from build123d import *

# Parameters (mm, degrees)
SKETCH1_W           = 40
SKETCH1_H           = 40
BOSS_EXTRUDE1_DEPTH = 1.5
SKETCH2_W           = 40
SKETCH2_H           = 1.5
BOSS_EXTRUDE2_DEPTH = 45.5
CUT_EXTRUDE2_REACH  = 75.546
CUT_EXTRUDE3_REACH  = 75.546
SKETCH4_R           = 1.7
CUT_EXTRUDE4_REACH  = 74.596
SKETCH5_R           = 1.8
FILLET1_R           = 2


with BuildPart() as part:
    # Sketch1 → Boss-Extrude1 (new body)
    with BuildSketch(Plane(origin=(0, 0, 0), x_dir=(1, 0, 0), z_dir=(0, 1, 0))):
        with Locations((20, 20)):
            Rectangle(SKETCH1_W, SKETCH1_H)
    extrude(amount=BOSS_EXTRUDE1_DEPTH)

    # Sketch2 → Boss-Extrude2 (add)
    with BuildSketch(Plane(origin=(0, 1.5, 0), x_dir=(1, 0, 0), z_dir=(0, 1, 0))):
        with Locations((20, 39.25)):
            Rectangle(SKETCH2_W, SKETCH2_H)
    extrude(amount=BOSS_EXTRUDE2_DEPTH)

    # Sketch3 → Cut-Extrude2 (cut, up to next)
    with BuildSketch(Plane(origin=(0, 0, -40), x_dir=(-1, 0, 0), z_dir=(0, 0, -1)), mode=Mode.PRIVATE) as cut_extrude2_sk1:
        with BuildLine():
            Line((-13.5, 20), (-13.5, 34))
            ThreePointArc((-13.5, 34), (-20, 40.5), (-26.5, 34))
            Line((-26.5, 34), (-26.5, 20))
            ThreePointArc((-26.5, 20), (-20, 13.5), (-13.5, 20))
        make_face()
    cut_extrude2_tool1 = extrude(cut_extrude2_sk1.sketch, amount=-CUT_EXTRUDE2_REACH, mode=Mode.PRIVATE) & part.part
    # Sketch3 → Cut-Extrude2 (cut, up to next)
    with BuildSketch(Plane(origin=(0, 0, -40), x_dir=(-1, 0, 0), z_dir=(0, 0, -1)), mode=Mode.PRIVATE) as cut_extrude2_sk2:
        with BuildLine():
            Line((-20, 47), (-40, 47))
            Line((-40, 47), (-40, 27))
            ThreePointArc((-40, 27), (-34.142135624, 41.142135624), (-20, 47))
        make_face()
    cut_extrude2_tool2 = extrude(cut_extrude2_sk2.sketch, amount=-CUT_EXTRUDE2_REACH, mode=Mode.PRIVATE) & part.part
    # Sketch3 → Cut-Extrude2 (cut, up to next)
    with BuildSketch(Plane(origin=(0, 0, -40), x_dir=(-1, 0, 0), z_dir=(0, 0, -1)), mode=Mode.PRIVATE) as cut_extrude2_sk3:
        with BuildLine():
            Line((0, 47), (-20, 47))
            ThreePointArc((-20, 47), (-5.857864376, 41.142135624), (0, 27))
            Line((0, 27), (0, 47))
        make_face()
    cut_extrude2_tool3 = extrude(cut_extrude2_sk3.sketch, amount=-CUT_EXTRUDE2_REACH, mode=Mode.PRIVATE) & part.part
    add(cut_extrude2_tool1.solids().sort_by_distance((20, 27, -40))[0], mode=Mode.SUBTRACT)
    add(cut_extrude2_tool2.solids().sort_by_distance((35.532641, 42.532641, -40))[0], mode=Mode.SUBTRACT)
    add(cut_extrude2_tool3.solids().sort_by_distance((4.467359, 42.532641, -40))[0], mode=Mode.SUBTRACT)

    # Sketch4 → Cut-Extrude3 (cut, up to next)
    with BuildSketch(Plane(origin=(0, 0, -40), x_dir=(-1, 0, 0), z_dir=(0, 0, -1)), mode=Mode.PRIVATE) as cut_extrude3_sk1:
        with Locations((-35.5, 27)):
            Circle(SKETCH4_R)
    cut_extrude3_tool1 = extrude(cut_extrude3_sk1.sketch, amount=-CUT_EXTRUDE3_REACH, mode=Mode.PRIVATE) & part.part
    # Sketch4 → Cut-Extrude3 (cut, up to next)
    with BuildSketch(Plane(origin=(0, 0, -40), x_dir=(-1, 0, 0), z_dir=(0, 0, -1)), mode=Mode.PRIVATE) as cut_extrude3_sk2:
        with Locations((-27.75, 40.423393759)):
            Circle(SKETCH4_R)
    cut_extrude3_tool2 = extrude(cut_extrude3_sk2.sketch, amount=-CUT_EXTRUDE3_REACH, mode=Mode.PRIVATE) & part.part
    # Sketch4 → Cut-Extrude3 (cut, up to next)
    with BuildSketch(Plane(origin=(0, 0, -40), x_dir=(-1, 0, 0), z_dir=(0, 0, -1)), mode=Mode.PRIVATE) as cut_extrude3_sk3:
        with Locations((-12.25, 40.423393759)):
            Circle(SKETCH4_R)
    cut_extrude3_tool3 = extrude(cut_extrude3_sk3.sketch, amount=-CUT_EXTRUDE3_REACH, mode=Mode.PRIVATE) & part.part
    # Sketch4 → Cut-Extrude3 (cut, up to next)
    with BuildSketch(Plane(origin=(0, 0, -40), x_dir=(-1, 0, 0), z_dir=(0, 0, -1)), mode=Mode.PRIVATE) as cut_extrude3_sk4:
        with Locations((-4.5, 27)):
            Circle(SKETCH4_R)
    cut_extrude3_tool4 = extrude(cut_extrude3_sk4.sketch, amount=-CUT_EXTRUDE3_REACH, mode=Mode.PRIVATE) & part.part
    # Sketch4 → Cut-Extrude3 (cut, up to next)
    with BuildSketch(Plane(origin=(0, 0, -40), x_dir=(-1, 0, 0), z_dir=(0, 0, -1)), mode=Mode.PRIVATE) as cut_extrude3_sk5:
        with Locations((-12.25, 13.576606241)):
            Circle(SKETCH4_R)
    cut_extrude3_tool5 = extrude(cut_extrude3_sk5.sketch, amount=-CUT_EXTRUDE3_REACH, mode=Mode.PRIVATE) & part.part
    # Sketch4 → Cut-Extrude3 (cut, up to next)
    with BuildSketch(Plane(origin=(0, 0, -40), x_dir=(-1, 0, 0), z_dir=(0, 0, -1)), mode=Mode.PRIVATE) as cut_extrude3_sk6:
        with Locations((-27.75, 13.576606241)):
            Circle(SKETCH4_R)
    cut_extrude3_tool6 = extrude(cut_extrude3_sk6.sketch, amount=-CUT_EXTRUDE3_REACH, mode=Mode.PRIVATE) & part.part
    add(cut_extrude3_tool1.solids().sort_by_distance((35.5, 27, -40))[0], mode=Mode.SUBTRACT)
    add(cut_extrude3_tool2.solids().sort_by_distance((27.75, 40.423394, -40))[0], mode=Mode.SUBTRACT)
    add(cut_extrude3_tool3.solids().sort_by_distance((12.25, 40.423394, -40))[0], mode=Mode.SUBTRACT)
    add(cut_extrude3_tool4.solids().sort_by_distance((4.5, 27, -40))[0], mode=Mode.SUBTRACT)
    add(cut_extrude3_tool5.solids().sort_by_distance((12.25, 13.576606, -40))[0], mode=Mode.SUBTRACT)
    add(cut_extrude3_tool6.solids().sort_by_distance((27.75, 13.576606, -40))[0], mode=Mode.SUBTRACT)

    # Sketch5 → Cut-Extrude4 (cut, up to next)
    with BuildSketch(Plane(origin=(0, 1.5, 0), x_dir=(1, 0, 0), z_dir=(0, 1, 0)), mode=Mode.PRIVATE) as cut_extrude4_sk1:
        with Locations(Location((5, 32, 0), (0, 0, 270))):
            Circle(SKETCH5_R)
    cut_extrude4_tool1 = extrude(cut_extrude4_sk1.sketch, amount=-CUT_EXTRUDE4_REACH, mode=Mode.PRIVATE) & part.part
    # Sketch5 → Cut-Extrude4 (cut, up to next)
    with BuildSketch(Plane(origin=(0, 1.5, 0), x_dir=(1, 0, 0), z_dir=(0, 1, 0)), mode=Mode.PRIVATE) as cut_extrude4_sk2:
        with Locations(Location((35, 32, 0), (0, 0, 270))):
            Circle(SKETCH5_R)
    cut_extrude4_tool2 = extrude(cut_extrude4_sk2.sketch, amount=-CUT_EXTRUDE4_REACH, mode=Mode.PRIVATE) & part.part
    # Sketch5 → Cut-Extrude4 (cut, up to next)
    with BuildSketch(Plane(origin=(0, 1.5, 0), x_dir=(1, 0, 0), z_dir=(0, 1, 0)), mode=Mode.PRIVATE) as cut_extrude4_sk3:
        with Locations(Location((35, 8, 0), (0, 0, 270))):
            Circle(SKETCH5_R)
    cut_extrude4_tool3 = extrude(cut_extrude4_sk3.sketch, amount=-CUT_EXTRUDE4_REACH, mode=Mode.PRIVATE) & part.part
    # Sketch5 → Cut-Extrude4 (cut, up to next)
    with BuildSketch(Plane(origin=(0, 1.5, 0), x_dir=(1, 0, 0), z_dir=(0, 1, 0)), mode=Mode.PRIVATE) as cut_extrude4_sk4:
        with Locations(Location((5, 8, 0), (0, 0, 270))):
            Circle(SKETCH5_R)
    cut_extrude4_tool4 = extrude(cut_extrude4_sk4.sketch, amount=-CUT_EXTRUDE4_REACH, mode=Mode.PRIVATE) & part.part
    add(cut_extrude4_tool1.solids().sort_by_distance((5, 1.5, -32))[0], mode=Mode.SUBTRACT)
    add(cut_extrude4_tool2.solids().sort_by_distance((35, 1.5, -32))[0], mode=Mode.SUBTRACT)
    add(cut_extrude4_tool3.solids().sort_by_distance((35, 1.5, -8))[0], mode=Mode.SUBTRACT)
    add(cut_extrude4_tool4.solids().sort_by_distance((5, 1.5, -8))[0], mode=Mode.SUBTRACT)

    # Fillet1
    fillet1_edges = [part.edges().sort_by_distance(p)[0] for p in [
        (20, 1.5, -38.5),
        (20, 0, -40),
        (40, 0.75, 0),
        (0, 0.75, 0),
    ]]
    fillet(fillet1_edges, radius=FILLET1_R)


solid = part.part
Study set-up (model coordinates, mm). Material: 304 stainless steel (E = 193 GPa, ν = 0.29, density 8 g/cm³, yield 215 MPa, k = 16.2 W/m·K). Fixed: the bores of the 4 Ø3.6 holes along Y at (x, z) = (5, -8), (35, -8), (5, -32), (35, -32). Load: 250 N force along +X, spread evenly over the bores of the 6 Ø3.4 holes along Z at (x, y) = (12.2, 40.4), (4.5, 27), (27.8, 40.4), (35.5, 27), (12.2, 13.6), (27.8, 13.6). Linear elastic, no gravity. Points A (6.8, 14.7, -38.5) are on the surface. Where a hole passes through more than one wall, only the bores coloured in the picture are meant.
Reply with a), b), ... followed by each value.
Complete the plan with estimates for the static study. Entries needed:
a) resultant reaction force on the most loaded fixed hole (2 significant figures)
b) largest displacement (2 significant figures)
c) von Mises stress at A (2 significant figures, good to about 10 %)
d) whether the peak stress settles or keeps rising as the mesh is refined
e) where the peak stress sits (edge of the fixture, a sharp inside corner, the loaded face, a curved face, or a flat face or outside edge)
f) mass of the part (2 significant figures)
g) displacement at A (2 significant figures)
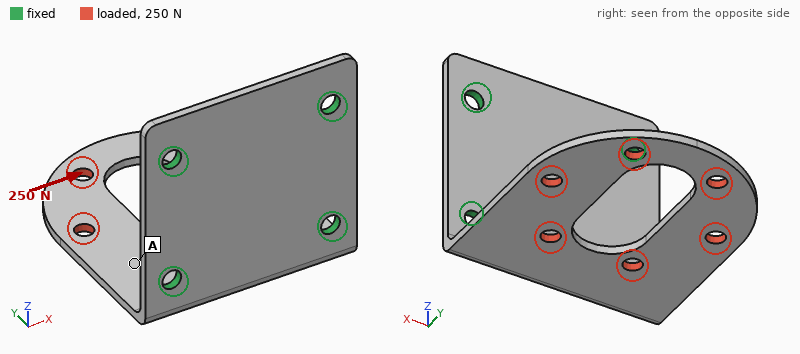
a) 250 N
b) 70 µm
c) 21 MPa
d) keeps rising
e) edge of the fixture
f) 34 g
g) 34 µm
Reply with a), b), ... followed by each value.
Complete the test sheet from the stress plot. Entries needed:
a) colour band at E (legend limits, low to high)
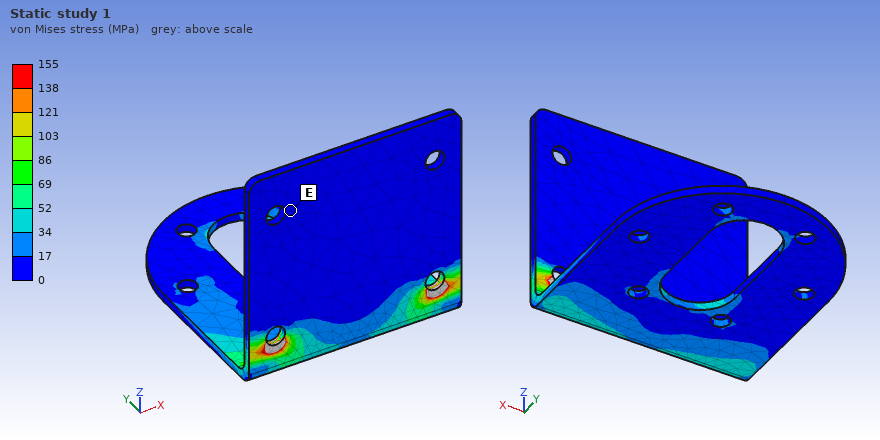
a) 0 to 17 MPa
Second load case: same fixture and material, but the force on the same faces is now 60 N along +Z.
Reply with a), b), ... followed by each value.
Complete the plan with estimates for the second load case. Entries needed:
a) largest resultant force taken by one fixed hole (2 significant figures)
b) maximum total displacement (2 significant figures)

a) 20 N
b) 0.61 mm
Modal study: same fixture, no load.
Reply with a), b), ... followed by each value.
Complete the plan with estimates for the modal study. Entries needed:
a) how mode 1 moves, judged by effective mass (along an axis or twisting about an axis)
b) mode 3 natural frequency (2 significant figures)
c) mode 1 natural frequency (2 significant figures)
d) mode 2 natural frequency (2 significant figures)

a) along Z
b) 3000 Hz
c) 610 Hz
d) 1600 Hz
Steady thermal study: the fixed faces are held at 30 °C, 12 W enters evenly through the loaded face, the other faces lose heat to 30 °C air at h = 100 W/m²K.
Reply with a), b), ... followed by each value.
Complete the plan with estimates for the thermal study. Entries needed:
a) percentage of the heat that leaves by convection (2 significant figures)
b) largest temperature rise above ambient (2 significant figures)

a) 93 %
b) 72 K
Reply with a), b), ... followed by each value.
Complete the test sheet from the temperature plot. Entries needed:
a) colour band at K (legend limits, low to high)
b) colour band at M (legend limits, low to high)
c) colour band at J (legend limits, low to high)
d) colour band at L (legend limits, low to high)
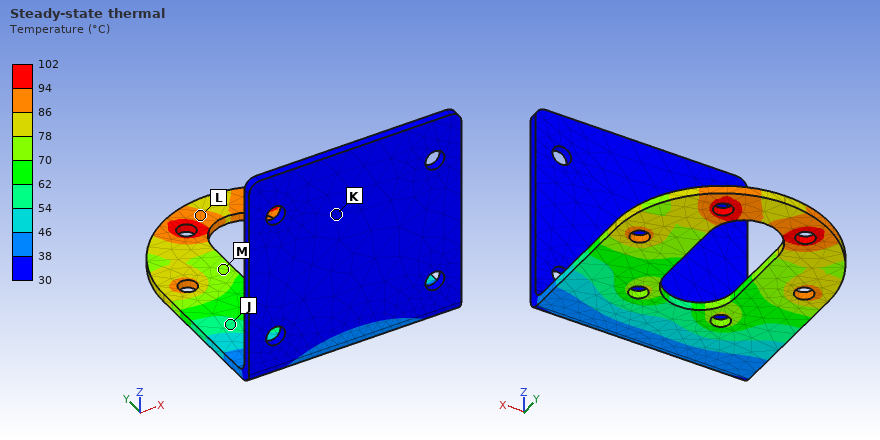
a) 30 to 38 °C
b) 70 to 78 °C
c) 54 to 62 °C
d) 86 to 94 °C
